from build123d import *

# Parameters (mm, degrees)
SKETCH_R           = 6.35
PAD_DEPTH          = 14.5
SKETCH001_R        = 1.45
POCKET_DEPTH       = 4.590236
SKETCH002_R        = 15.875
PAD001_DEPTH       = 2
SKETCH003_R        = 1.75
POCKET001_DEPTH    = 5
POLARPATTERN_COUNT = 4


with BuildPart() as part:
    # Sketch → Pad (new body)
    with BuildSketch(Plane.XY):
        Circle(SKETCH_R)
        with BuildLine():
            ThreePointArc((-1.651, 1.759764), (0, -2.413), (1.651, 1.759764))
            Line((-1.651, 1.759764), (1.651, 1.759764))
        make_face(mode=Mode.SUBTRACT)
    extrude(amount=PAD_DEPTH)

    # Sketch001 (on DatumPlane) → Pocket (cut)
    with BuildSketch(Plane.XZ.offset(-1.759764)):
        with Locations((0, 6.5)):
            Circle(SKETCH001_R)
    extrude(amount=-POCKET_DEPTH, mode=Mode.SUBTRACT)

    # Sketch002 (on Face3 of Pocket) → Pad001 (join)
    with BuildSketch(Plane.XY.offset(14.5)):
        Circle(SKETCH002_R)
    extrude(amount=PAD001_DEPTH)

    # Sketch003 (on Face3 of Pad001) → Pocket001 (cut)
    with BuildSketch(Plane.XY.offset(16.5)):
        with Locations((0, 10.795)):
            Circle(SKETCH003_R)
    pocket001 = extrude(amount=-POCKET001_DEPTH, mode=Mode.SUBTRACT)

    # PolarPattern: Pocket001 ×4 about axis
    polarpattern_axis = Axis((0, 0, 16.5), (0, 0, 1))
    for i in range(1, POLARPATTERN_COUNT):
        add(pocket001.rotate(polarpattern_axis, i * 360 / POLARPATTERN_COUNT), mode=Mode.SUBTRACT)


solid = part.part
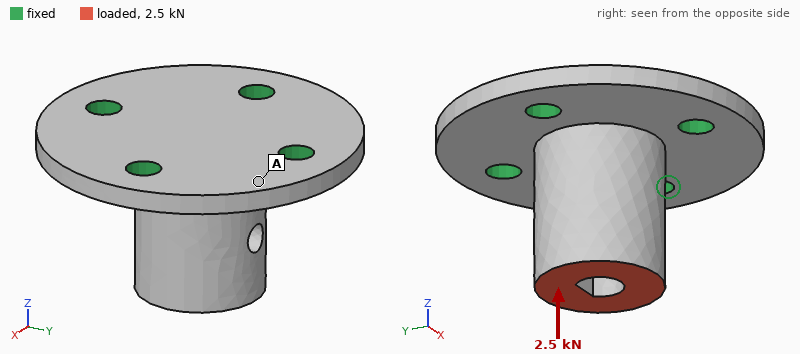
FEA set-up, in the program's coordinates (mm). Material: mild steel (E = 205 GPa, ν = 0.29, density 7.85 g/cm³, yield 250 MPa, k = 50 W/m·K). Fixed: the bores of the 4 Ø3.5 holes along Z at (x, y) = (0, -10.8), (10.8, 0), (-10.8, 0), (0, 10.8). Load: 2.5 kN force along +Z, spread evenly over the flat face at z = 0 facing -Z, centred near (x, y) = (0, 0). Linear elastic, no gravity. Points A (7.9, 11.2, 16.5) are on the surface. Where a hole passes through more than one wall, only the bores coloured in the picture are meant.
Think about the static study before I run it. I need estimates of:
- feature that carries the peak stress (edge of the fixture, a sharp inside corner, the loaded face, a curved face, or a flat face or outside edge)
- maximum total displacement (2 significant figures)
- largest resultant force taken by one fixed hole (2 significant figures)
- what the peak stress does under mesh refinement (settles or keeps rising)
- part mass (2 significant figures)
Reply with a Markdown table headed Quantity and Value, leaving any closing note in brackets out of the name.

| Quantity | Value |
|---|---|
| feature that carries the peak stress | edge of the fixture |
| maximum total displacement | 8.1 µm |
| largest resultant force taken by one fixed hole | 660 N |
| what the peak stress does under mesh refinement | keeps rising |
| part mass | 24 g |
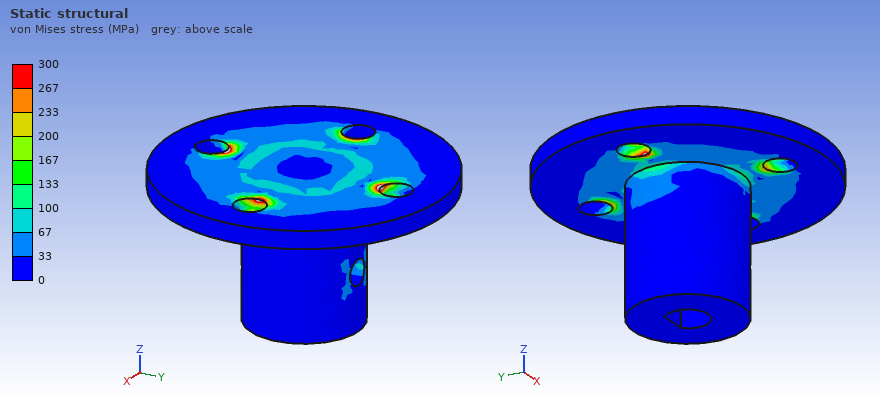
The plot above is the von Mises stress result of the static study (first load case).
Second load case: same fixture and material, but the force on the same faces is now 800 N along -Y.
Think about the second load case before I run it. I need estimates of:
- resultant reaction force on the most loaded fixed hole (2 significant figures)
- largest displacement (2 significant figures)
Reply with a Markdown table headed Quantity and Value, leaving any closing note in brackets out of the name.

| Quantity | Value |
|---|---|
| resultant reaction force on the most loaded fixed hole | 760 N |
| largest displacement | 20 µm |
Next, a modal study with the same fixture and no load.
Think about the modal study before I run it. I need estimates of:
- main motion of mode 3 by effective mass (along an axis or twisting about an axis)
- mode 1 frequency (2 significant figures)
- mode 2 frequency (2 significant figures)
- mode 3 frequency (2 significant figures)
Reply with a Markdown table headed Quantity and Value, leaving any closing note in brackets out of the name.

| Quantity | Value |
|---|---|
| main motion of mode 3 by effective mass | along Z |
| mode 1 frequency | 15 kHz |
| mode 2 frequency | 15 kHz |
| mode 3 frequency | 25 kHz |
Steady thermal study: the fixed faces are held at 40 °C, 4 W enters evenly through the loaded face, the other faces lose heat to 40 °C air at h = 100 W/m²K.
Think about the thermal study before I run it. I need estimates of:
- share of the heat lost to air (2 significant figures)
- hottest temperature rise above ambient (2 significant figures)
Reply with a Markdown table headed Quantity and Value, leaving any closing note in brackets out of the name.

| Quantity | Value |
|---|---|
| share of the heat lost to air | 23 % |
| hottest temperature rise above ambient | 14 K |
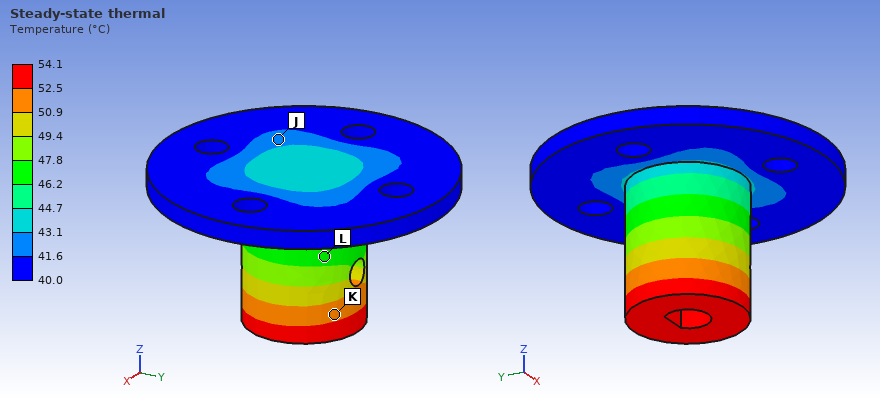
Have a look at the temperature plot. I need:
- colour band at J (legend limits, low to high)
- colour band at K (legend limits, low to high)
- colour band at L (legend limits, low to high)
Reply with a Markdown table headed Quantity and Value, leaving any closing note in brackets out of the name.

| Quantity | Value |
|---|---|
| colour band at J | 41.6 to 43.1 °C |
| colour band at K | 50.9 to 52.5 °C |
| colour band at L | 46.2 to 47.8 °C |
